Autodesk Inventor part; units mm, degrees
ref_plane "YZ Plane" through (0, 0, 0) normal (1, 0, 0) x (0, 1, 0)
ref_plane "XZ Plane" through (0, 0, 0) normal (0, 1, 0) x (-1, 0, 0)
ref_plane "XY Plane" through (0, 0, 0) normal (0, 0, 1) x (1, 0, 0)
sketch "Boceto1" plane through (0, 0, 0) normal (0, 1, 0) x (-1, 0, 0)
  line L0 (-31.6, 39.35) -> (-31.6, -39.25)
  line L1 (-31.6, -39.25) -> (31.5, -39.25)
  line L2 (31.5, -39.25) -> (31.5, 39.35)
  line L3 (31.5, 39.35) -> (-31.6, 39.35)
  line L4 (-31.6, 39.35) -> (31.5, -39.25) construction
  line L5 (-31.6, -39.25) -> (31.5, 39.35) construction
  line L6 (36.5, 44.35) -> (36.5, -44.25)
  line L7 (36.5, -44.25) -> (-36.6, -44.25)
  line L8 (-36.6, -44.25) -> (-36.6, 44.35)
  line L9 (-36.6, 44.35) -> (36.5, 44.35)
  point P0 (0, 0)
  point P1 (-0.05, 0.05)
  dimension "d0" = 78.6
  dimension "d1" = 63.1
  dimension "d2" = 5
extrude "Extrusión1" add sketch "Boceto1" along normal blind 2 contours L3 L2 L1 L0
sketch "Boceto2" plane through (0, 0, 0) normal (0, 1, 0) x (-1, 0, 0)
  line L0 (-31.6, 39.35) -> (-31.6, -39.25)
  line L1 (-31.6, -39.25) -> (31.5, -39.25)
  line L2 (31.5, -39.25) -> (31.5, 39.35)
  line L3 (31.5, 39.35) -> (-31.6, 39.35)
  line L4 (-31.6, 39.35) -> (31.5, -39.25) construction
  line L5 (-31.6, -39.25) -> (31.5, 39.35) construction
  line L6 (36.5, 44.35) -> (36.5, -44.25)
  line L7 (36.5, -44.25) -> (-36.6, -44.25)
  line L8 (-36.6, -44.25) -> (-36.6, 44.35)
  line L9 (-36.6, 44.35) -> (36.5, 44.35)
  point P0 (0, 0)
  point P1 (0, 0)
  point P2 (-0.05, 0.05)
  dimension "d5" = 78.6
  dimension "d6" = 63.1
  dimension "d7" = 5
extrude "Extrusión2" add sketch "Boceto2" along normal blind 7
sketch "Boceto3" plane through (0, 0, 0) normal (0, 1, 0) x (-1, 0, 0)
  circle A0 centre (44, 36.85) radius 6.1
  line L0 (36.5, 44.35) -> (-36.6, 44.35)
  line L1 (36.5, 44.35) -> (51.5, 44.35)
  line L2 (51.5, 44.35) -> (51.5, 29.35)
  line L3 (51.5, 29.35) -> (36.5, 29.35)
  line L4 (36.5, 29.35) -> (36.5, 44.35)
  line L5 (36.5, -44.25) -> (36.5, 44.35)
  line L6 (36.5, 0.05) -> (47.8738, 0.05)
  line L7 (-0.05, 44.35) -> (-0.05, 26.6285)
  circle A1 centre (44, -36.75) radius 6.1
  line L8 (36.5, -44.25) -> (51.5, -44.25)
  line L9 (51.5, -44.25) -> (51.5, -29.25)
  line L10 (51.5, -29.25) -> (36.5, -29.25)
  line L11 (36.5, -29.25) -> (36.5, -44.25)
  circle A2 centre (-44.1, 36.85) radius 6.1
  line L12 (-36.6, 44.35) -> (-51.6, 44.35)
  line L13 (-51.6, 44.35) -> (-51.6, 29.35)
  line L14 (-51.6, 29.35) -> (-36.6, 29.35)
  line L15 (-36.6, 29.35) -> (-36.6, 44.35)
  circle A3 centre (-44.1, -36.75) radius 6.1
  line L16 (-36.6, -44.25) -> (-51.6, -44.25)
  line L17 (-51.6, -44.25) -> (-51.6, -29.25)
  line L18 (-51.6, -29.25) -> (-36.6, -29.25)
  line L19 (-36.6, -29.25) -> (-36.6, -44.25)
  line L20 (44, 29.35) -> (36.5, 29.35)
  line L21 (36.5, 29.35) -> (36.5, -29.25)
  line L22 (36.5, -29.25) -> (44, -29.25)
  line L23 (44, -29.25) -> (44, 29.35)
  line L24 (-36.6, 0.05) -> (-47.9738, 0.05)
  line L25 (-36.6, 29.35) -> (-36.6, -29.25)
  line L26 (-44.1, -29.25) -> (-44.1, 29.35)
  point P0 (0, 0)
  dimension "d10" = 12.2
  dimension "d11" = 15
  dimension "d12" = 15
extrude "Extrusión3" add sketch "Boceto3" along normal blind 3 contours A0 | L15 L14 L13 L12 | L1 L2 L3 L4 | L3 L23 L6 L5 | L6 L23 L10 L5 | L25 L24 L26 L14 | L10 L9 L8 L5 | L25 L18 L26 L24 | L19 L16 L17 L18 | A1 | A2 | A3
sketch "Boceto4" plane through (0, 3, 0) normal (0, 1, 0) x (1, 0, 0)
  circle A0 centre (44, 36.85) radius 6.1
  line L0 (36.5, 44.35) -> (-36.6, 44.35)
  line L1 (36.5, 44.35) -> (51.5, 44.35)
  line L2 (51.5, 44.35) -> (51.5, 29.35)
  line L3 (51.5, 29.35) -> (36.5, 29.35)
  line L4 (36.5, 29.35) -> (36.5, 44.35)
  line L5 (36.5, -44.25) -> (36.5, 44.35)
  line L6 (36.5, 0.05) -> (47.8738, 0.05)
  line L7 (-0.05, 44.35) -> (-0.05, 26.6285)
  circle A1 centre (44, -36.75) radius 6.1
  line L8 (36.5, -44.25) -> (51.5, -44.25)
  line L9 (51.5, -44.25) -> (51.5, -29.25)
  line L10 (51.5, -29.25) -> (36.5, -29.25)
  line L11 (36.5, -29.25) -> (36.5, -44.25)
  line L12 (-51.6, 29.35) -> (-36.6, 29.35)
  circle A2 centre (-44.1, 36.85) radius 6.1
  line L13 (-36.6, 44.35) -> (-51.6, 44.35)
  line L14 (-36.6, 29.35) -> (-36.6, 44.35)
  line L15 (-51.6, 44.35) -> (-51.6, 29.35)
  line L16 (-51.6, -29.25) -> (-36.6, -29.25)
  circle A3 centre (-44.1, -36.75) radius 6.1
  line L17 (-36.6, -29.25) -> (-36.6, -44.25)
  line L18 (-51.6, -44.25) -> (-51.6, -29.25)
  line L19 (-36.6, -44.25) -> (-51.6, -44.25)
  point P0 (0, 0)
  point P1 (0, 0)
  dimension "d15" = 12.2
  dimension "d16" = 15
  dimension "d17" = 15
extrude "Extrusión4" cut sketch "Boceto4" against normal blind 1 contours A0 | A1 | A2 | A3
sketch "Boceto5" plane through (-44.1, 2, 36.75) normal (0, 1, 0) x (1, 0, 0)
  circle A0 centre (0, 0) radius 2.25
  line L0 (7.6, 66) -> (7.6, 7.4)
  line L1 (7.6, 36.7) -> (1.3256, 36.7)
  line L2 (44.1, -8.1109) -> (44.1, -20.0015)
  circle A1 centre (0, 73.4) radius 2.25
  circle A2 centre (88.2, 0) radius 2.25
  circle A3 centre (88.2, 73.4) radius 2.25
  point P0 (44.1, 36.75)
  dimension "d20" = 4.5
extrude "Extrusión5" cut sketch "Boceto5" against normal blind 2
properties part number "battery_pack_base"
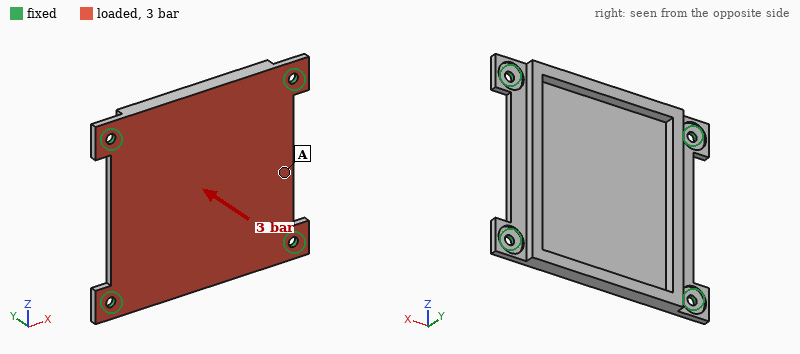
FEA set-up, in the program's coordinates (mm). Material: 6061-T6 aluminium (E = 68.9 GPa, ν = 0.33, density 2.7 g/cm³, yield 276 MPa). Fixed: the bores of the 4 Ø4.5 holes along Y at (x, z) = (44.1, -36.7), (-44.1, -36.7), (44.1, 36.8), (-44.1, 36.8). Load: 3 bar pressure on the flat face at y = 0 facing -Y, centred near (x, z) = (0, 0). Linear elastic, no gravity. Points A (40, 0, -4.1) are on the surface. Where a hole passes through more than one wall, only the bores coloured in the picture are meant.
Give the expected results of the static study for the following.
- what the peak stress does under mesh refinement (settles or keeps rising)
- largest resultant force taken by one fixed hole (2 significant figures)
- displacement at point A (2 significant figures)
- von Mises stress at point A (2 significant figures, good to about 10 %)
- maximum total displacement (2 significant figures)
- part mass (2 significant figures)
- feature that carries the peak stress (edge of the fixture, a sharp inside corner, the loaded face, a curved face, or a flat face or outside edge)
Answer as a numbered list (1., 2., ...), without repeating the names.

1. keeps rising
2. 1.0 kN
3. 0.15 mm
4. 30 MPa
5. 0.65 mm
6. 68 g
7. edge of the fixture
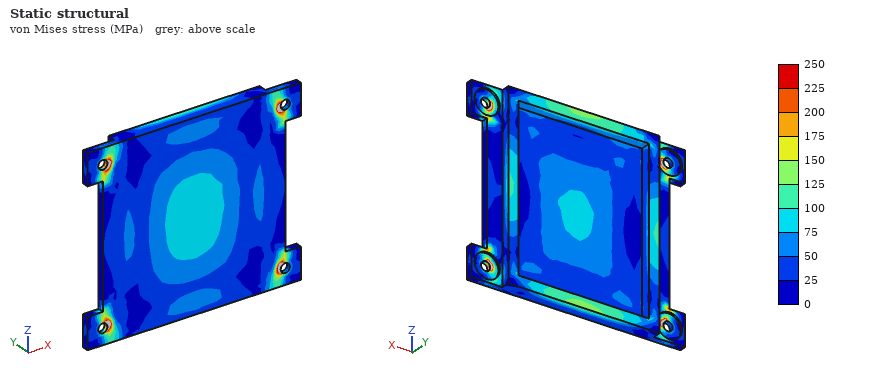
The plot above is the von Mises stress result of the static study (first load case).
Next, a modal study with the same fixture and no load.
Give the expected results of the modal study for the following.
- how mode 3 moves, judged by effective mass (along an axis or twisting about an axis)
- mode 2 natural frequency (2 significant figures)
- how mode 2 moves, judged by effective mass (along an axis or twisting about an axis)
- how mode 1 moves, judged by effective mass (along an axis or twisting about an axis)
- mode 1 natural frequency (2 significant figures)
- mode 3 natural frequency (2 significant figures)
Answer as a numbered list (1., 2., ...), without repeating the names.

1. twisting about Z
2. 2900 Hz
3. twisting about X
4. along Y
5. 1800 Hz
6. 3300 Hz
